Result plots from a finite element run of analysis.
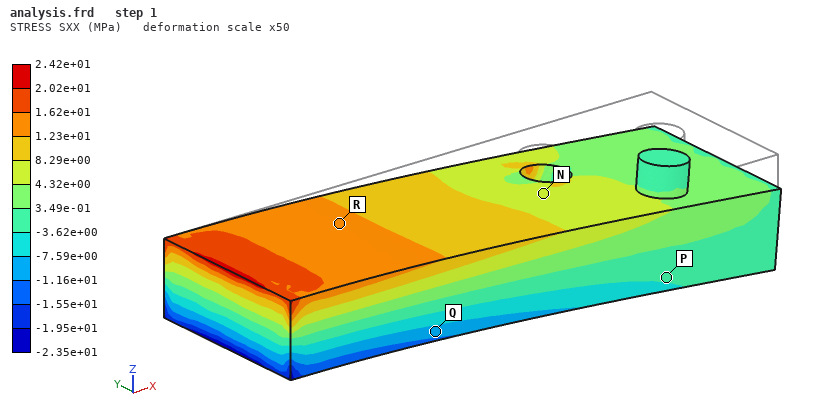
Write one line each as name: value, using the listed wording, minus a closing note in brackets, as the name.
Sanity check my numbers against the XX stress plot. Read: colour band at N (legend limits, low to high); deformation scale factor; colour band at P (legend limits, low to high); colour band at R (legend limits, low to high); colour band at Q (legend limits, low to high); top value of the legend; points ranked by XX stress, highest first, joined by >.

colour band at N: 4.32e+00 to 8.29e+00 MPa
deformation scale factor: 50
colour band at P: -3.62e+00 to 3.49e-01 MPa
colour band at R: 1.23e+01 to 1.62e+01 MPa
colour band at Q: -1.16e+01 to -7.59e+00 MPa
top value of the legend: 2.42e+01 MPa
points ranked by XX stress, highest first, joined by >: R > N > P > Q
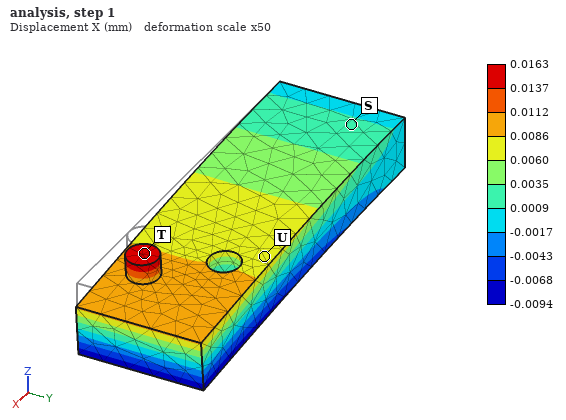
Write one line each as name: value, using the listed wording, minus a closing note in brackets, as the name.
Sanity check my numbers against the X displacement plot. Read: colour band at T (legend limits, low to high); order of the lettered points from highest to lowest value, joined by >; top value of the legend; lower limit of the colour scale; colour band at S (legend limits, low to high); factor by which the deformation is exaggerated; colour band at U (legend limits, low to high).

colour band at T: 0.0137 to 0.0163 mm
order of the lettered points from highest to lowest value, joined by >: T > U > S
top value of the legend: 0.0163 mm
lower limit of the colour scale: -0.0094 mm
colour band at S: 0.0009 to 0.0035 mm
factor by which the deformation is exaggerated: 50
colour band at U: 0.0060 to 0.0086 mm
